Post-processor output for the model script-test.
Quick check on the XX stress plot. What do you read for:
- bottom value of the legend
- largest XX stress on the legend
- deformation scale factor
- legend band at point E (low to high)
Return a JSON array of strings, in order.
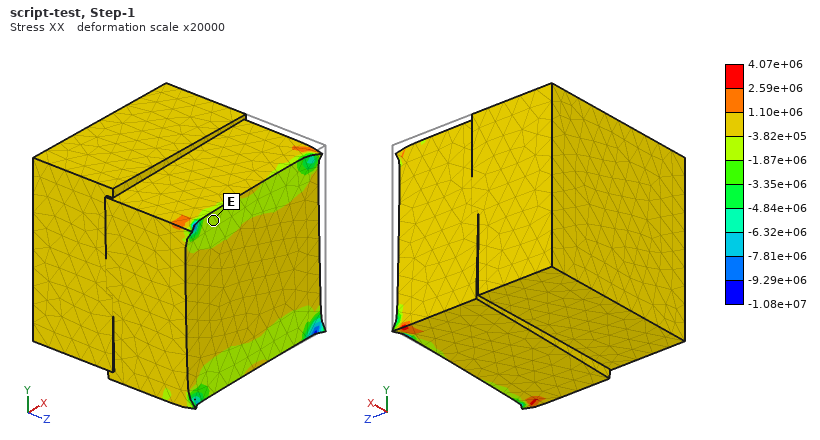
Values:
["-1.08e+07", "4.07e+06", "20000", "-1.87e+06 to -3.82e+05"]
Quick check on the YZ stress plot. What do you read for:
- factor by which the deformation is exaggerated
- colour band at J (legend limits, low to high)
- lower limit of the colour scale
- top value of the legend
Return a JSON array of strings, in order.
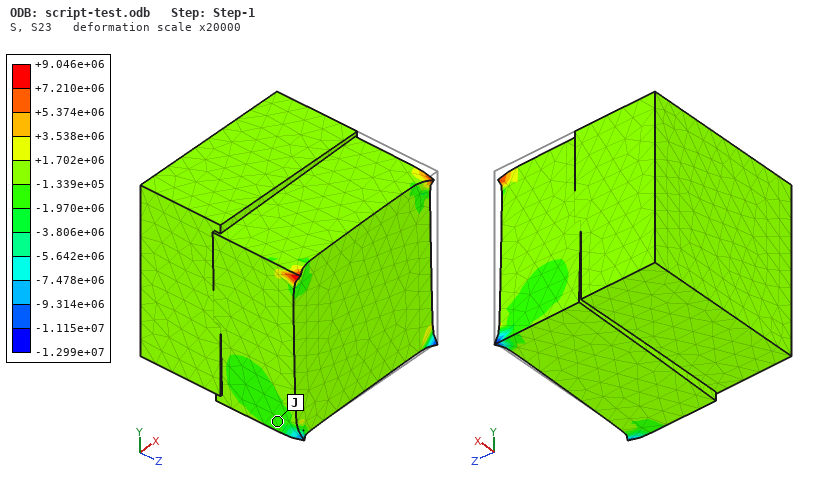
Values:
["20000", "-1.970e+06 to -1.339e+05", "-1.299e+07", "+9.046e+06"]
